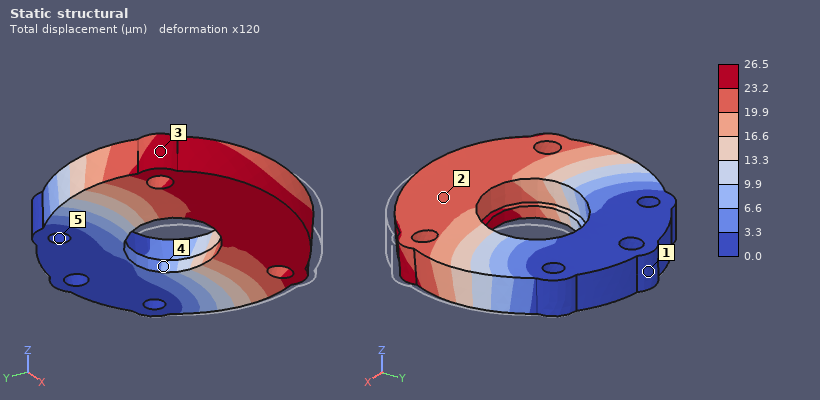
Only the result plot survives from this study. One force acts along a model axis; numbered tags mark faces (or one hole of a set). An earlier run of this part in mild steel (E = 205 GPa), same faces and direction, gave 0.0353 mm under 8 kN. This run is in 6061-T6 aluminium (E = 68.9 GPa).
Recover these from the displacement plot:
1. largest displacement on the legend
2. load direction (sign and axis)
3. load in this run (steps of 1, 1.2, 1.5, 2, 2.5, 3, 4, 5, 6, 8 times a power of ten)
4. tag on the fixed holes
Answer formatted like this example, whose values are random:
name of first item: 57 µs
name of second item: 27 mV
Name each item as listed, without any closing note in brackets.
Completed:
largest displacement on the legend: 26.5 µm
load direction: -X
load in this run: 2 kN
tag on the fixed holes: 5
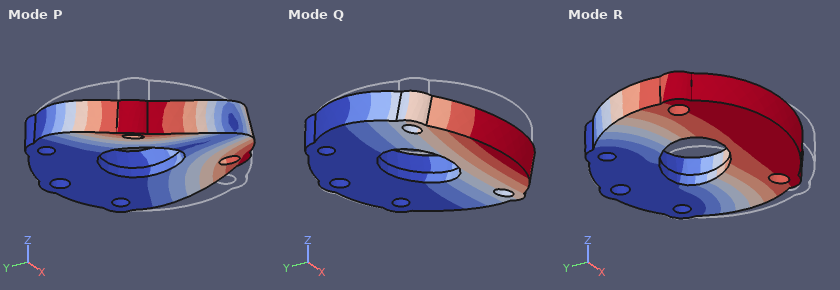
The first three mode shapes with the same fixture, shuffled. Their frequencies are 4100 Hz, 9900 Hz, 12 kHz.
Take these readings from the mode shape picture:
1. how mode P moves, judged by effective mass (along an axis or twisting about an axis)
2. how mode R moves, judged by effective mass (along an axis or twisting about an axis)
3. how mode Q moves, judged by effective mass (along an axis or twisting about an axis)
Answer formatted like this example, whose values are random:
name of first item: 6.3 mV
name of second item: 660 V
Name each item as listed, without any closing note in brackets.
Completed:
how mode P moves, judged by effective mass: twisting about Y
how mode R moves, judged by effective mass: along X
how mode Q moves, judged by effective mass: along Z
